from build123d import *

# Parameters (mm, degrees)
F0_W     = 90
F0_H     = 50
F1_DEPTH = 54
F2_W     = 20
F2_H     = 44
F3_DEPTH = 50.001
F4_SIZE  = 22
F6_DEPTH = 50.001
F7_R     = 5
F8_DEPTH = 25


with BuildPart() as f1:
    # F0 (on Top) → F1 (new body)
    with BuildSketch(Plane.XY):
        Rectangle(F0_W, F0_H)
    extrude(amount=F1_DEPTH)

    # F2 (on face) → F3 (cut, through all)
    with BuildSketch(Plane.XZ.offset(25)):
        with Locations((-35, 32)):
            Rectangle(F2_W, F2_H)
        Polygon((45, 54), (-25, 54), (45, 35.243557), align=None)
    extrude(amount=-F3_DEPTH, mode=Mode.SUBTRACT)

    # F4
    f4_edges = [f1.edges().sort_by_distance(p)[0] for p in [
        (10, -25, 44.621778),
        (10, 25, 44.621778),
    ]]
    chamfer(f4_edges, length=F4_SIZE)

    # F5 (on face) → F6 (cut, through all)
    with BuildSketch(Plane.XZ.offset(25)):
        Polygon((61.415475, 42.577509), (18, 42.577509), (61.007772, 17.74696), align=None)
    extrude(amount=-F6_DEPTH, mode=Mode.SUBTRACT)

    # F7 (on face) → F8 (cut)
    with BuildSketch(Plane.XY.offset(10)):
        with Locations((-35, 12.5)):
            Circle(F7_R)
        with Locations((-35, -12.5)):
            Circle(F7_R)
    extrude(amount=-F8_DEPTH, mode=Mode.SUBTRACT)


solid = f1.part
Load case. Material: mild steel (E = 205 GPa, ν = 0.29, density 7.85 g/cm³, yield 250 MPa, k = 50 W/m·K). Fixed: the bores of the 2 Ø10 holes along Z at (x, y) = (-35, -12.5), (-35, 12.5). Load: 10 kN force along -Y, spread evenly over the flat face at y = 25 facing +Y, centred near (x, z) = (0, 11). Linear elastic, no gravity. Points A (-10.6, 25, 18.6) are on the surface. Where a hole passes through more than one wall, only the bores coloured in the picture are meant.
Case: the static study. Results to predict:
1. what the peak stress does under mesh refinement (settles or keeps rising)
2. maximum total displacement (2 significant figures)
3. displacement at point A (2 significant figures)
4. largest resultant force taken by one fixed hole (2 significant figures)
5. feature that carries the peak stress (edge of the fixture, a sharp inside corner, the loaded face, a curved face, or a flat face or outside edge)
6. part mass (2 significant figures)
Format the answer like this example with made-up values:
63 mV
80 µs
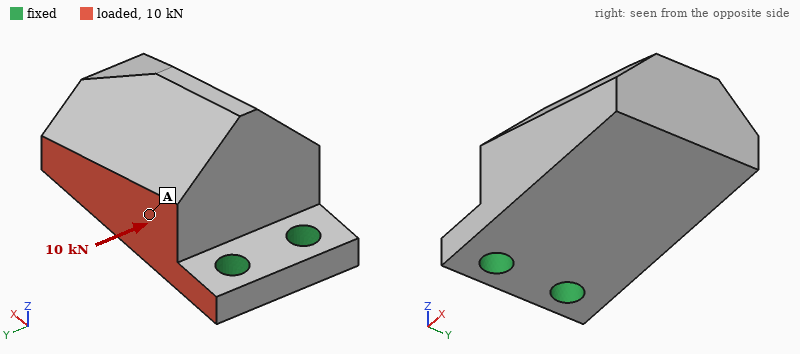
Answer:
keeps rising
32 µm
13 µm
12 kN
edge of the fixture
1.0 kg
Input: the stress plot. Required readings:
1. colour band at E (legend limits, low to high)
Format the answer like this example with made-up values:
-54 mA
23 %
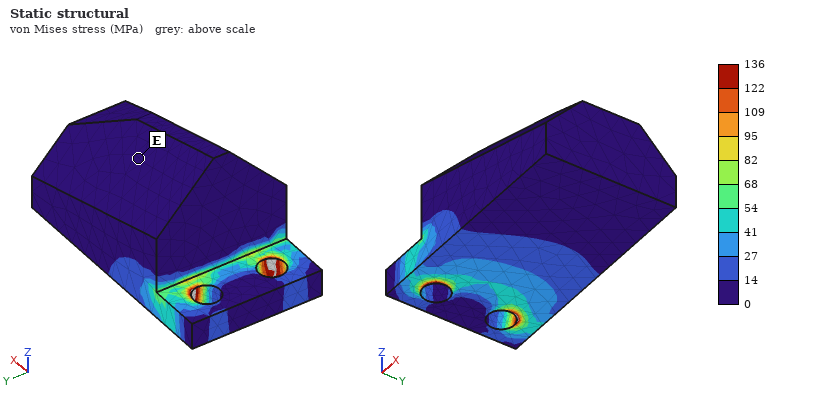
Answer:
0 to 14 MPa
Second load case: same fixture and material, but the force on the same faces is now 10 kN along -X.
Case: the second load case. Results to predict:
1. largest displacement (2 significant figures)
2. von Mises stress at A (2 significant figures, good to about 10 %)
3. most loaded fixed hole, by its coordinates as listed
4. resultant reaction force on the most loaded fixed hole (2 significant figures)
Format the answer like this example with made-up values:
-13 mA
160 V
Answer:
64 µm
16 MPa
(-35, 12.5)
13 kN
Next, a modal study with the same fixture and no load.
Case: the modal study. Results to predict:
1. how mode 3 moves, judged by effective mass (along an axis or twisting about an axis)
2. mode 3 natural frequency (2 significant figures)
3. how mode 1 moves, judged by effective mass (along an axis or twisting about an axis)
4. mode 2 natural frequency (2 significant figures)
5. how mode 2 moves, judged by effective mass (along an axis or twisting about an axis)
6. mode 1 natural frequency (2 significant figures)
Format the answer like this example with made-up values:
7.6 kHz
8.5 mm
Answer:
twisting about X
4700 Hz
along Z
3300 Hz
along Y
1000 Hz
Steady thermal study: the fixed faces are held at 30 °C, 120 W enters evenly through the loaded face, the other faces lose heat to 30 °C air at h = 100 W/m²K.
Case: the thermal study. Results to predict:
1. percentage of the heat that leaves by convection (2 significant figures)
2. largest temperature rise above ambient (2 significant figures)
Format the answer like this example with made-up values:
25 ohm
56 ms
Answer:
43 %
66 K
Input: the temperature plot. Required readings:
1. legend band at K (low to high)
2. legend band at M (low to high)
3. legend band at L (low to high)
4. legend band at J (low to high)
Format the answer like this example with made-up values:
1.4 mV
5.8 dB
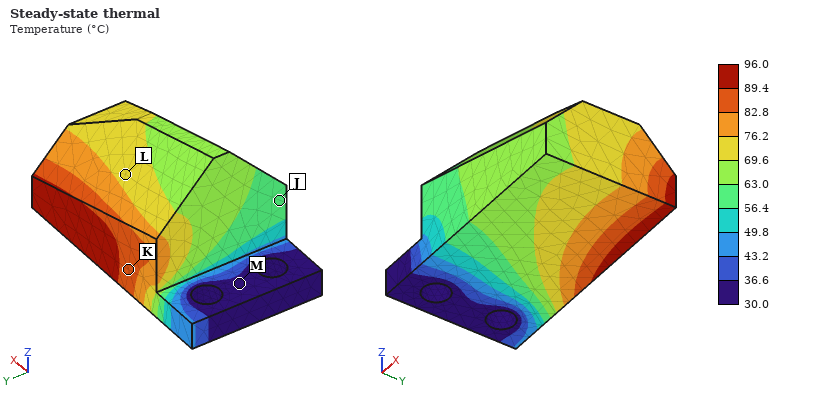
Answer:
82.8 to 89.4 °C
30.0 to 36.6 °C
69.6 to 76.2 °C
56.4 to 63.0 °C
